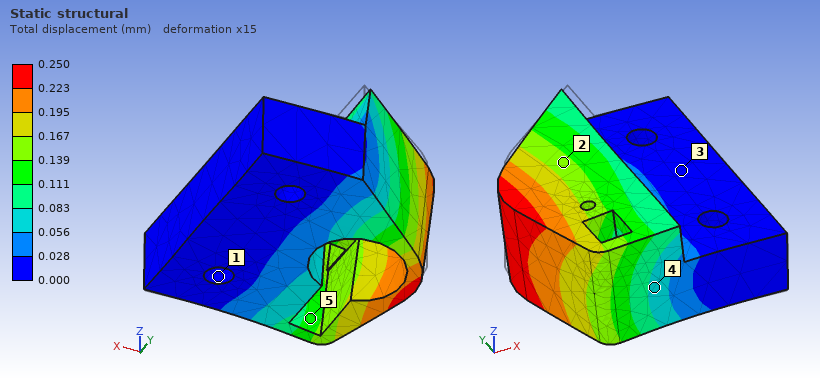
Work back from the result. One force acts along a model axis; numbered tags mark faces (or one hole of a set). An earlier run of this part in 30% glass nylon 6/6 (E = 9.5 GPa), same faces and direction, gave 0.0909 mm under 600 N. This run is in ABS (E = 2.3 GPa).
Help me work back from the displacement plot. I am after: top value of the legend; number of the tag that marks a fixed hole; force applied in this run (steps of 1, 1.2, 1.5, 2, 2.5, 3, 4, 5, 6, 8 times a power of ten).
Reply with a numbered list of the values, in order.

1. 0.250 mm
2. 1
3. 400 N
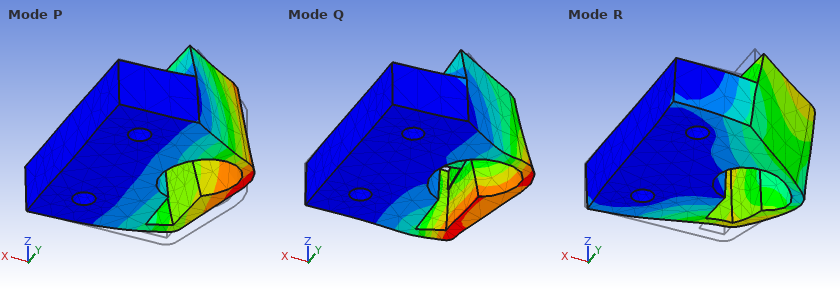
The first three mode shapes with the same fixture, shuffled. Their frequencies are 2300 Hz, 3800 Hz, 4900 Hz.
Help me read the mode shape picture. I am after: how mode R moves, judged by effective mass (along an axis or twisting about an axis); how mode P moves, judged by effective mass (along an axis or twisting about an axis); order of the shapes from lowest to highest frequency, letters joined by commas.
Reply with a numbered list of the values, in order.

1. along Y
2. along Z
3. P, Q, R
